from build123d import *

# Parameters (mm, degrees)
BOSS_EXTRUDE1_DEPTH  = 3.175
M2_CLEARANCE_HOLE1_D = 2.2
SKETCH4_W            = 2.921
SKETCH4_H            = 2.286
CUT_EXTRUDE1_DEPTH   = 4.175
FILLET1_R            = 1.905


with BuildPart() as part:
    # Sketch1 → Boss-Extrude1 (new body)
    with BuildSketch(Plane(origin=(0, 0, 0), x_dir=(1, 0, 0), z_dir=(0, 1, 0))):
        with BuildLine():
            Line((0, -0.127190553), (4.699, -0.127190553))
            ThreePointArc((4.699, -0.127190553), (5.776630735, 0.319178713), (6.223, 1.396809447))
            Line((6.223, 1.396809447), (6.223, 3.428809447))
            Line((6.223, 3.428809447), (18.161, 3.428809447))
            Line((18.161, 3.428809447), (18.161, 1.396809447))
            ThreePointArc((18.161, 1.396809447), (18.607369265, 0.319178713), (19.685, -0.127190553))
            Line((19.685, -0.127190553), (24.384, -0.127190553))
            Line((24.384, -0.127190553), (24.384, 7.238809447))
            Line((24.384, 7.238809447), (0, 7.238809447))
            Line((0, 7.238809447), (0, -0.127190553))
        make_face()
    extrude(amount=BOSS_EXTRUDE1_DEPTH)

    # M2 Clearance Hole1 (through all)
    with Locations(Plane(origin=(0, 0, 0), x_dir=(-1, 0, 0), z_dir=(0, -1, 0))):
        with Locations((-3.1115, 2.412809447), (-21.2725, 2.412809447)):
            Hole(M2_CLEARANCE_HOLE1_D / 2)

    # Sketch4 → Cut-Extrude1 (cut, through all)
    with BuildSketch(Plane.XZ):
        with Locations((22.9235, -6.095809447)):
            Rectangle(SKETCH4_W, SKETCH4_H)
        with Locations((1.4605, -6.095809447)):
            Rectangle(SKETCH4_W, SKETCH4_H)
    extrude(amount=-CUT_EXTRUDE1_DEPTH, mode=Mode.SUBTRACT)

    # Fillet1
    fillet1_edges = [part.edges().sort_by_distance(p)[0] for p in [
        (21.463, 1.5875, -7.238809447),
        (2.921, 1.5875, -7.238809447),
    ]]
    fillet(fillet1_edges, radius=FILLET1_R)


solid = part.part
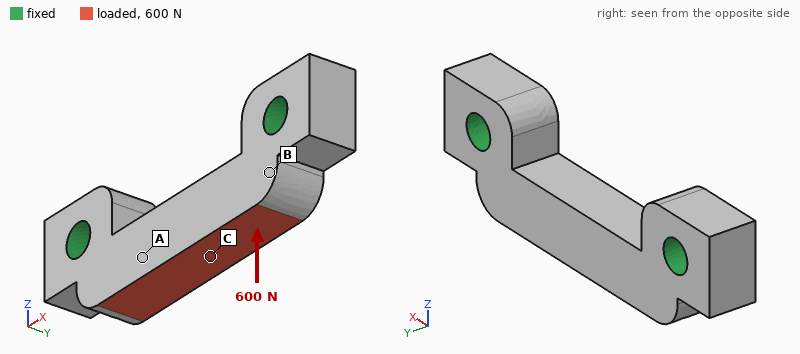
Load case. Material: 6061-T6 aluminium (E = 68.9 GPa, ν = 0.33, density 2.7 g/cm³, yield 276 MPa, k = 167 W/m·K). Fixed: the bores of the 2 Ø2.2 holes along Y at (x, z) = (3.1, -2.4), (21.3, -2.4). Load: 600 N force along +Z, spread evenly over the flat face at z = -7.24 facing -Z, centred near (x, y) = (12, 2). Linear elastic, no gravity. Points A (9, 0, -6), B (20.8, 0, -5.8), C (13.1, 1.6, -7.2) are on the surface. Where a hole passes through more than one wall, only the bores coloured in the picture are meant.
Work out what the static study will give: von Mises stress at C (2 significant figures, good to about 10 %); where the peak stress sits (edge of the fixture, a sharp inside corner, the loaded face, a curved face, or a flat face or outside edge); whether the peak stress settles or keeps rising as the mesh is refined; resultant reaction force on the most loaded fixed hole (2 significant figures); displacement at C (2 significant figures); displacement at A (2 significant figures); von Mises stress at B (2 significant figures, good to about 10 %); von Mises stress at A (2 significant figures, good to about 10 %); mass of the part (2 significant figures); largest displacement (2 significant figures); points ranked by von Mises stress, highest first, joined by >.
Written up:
74 MPa
edge of the fixture
keeps rising
380 N
12 µm
9.5 µm
11 MPa
39 MPa
0.97 g
12 µm
C > A > B
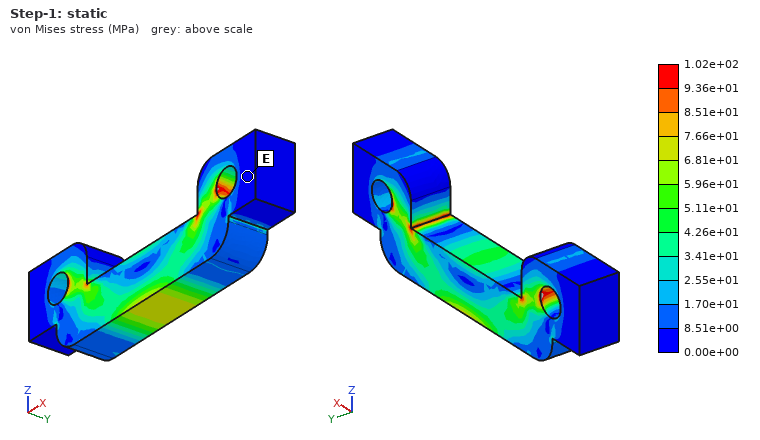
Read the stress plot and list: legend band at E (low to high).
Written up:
0.00e+00 to 8.51e+00 MPa
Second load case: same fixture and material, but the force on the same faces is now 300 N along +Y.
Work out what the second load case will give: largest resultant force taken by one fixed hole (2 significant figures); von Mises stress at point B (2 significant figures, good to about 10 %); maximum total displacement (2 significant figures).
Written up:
150 N
47 MPa
22 µm
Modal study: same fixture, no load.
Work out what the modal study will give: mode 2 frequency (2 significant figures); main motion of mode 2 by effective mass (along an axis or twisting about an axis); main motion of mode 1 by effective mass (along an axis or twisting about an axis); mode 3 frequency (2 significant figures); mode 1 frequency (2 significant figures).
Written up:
56 kHz
along Z
along Y
80 kHz
40 kHz
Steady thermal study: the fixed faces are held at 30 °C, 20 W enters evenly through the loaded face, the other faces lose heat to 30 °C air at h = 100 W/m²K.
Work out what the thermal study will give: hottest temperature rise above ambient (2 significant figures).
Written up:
30 K
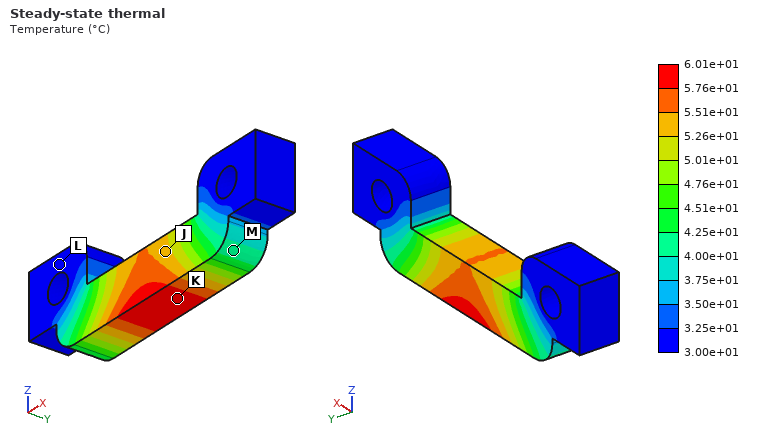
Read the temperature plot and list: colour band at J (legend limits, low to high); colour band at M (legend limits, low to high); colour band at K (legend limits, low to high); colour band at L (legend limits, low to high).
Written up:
5.26e+01 to 5.51e+01 °C
4.00e+01 to 4.25e+01 °C
5.76e+01 to 6.01e+01 °C
3.00e+01 to 3.25e+01 °C
